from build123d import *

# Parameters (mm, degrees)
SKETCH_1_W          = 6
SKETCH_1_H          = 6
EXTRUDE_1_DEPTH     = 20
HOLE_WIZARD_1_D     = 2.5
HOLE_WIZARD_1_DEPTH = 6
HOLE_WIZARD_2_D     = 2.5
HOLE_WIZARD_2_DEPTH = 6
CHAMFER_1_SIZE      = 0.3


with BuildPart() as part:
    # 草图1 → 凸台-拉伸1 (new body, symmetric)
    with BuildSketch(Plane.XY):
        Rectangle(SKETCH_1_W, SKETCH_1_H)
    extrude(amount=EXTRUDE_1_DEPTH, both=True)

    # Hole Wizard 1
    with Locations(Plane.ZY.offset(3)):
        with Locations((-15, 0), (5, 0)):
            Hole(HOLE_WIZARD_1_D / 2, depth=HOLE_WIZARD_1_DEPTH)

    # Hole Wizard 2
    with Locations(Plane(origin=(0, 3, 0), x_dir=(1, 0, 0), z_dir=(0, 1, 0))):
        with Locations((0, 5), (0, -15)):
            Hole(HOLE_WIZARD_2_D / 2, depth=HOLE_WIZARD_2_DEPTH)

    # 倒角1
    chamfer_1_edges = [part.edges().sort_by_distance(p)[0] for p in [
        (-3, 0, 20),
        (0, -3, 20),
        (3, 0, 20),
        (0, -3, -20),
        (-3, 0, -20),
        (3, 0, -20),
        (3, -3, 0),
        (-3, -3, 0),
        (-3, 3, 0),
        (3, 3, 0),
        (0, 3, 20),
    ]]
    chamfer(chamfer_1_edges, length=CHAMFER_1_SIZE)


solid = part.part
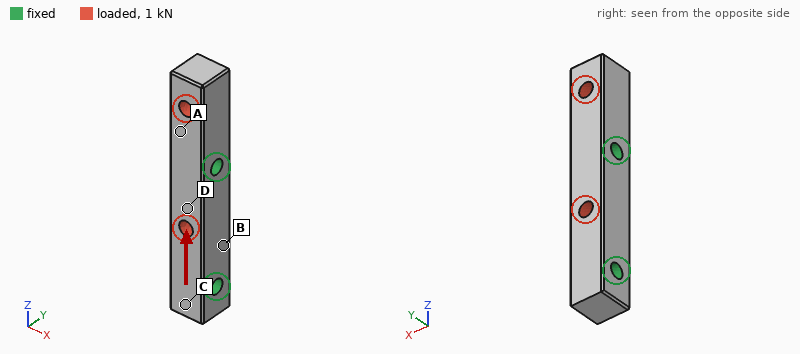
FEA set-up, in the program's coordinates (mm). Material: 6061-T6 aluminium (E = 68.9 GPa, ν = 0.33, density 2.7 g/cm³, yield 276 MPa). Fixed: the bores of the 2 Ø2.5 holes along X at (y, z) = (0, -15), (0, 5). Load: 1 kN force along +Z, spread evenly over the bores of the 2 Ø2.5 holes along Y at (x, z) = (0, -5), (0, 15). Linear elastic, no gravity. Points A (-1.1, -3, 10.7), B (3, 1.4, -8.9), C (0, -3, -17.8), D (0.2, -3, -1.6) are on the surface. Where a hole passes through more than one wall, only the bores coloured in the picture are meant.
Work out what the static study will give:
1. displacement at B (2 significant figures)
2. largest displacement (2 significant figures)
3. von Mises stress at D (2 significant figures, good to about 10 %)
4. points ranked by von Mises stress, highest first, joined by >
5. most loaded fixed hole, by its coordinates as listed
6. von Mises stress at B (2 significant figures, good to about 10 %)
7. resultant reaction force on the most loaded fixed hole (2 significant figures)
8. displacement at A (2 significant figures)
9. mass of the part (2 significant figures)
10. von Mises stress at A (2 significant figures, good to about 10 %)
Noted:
0.63 µm
2.7 µm
8.8 MPa
A > D > B > C
(0, 5)
6.3 MPa
740 N
1.2 µm
3.5 g
13 MPa
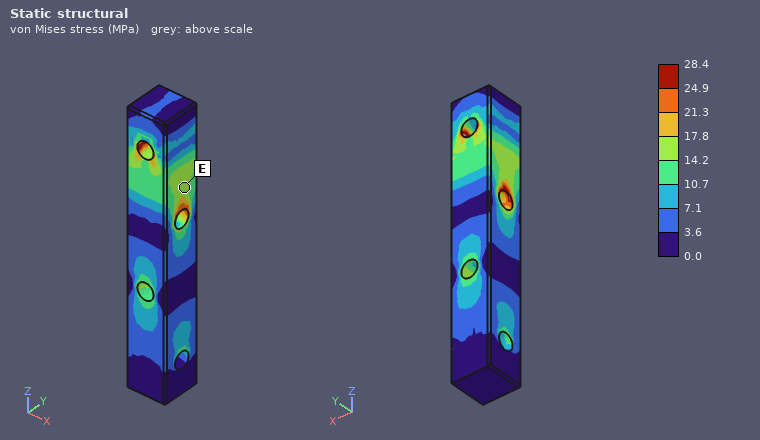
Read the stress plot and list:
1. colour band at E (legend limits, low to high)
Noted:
14.2 to 17.8 MPa
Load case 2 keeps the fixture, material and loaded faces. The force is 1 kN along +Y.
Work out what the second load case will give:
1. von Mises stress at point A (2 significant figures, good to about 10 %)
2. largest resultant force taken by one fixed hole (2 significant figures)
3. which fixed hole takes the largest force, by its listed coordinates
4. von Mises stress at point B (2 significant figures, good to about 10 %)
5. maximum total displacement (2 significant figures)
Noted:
60 MPa
810 N
(0, 5)
13 MPa
54 µm
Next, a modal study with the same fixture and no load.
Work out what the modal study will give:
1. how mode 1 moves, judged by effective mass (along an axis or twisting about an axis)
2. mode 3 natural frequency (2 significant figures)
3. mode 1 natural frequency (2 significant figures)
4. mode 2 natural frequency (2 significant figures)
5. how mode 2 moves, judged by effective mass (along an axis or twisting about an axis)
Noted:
along Y
49 kHz
18 kHz
21 kHz
along X
